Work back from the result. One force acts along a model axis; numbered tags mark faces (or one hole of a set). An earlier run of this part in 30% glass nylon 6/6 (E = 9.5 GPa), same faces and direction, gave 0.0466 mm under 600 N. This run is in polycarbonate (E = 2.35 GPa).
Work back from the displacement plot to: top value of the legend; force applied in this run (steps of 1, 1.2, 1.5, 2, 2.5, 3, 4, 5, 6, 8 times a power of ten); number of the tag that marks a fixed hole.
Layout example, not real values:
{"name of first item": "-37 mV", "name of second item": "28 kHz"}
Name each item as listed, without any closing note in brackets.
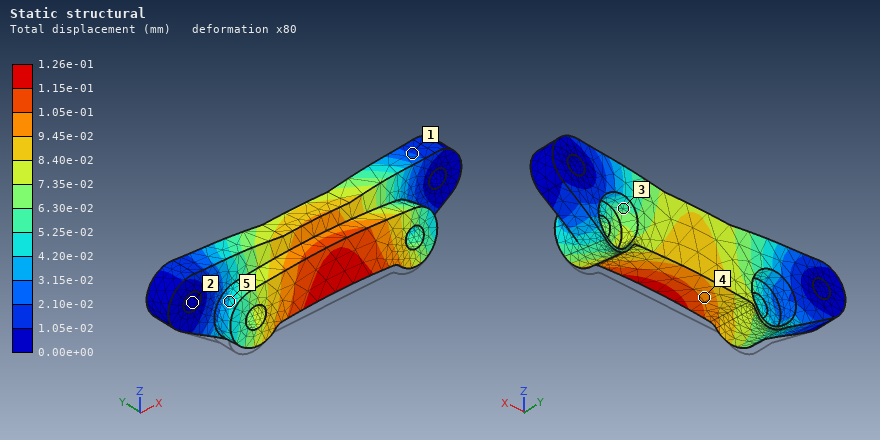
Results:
{"top value of the legend": "1.26e-01 mm", "force applied in this run": "400 N", "number of the tag that marks a fixed hole": "2"}
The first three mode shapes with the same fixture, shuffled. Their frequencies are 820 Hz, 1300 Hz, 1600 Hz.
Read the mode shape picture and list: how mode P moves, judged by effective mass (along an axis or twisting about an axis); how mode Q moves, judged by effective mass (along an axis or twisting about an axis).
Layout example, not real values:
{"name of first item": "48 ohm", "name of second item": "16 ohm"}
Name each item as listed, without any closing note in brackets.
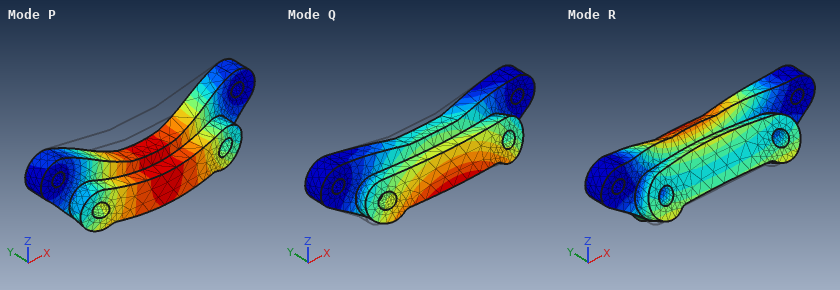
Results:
{"how mode P moves, judged by effective mass": "along Z", "how mode Q moves, judged by effective mass": "along Y"}
